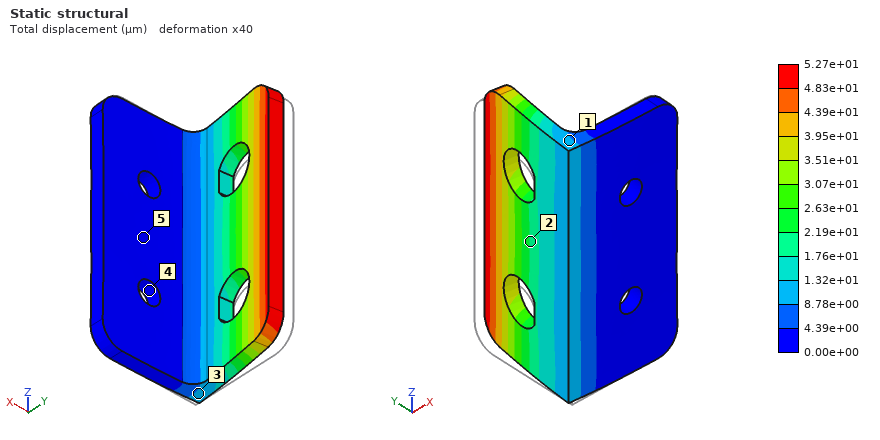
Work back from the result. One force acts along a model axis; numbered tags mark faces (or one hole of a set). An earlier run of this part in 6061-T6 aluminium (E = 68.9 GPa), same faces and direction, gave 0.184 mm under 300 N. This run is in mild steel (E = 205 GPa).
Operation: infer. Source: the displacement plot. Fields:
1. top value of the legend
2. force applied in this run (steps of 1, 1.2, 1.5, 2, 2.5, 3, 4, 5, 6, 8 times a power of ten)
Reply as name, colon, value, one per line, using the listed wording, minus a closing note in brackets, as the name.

top value of the legend: 5.27e+01 µm
force applied in this run: 250 N
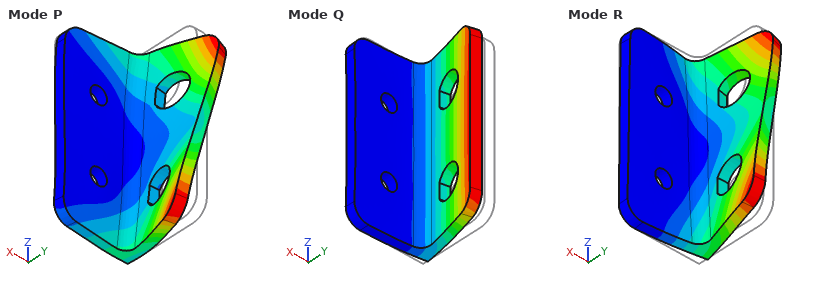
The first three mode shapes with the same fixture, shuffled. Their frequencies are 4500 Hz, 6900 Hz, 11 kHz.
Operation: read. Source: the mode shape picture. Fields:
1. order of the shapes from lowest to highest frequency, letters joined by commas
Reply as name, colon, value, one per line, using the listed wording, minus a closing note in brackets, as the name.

order of the shapes from lowest to highest frequency, letters joined by commas: Q, R, P
